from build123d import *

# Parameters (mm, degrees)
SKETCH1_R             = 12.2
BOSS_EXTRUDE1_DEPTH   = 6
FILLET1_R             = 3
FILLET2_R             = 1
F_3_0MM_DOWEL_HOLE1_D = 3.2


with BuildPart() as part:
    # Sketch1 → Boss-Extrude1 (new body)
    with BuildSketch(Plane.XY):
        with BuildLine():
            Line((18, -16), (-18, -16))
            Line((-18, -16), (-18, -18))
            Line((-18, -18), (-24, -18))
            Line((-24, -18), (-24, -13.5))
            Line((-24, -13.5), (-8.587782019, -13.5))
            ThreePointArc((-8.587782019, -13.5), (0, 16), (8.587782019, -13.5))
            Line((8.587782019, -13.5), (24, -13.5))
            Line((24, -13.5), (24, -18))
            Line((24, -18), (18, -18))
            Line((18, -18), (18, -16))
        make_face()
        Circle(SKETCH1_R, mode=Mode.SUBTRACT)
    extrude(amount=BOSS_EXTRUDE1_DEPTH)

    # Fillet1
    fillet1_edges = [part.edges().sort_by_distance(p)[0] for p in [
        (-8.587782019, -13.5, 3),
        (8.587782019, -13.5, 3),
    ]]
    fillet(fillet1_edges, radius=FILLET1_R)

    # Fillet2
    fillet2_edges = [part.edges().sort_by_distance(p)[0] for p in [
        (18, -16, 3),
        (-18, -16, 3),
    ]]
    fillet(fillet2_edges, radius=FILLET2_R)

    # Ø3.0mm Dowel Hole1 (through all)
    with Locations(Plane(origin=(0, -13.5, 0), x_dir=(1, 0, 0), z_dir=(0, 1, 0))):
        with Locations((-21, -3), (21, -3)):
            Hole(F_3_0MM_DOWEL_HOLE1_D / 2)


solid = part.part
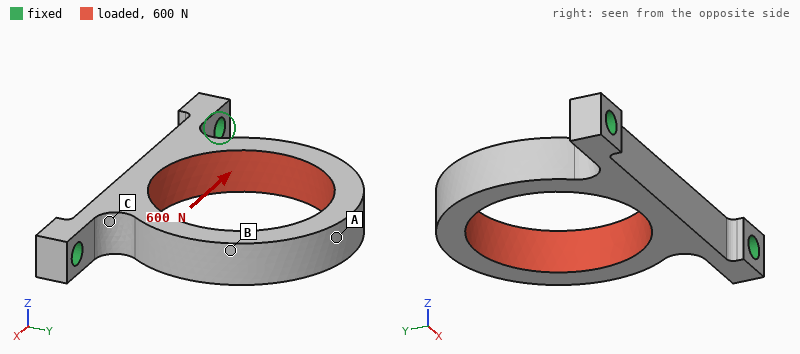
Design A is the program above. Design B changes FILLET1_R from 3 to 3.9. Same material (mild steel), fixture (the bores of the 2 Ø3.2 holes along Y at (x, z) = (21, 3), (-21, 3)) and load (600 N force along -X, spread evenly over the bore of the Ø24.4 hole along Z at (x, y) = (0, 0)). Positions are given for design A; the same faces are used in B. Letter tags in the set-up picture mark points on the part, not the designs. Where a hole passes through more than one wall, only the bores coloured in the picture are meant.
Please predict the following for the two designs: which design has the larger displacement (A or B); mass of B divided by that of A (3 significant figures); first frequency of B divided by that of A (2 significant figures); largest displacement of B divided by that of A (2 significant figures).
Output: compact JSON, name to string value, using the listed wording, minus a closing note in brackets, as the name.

{"which design has the larger displacement": "A", "mass of B divided by that of A": "1.02", "first frequency of B divided by that of A": "1.1", "largest displacement of B divided by that of A": "0.82"}
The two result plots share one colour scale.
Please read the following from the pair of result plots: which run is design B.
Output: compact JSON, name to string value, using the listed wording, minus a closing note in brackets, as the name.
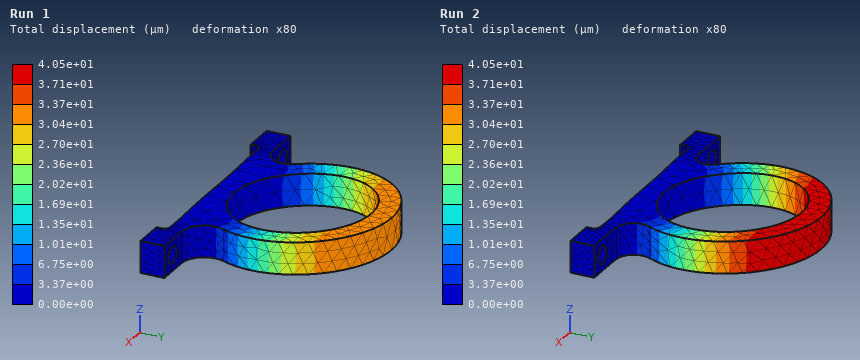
{"which run is design B": "Run 1"}
